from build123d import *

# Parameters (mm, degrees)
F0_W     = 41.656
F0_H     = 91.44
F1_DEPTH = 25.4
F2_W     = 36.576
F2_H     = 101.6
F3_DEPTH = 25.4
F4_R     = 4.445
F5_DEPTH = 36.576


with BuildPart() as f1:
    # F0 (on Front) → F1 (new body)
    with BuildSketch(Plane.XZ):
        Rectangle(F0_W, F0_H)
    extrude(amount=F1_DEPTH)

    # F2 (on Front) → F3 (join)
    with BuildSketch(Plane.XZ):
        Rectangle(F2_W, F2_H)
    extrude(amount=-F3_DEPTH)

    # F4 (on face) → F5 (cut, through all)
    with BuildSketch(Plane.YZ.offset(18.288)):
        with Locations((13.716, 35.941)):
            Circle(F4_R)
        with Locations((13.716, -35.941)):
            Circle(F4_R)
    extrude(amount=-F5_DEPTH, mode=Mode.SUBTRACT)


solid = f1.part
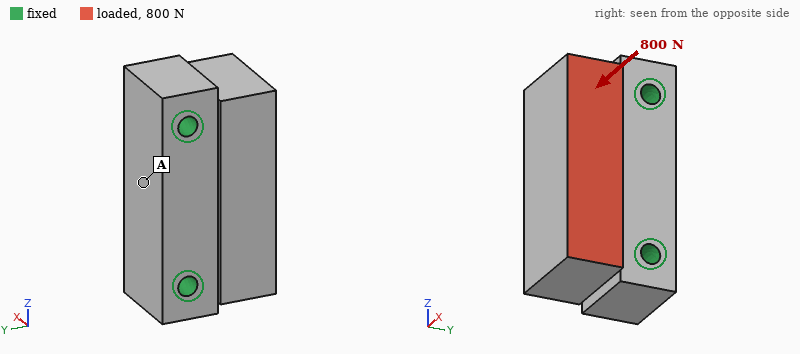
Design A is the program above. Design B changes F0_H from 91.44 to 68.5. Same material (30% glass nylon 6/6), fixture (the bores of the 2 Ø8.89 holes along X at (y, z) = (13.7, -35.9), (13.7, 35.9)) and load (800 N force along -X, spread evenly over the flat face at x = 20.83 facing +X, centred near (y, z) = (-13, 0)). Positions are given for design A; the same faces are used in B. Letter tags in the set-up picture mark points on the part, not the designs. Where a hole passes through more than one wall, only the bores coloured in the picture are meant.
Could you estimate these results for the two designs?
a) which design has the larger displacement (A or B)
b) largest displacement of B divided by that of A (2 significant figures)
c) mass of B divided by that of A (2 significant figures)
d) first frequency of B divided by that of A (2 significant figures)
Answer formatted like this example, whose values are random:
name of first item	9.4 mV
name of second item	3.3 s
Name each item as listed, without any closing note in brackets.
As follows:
which design has the larger displacement	B
largest displacement of B divided by that of A	1.5
mass of B divided by that of A	0.87
first frequency of B divided by that of A	0.93
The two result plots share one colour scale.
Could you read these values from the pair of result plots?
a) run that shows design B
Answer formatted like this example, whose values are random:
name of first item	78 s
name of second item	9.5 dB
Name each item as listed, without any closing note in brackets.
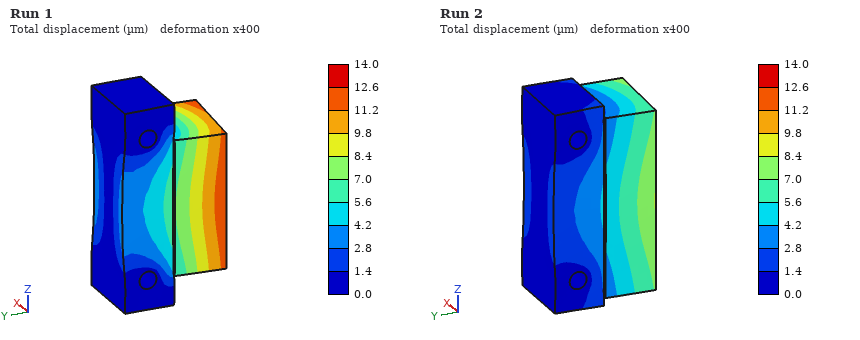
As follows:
run that shows design B	Run 1
